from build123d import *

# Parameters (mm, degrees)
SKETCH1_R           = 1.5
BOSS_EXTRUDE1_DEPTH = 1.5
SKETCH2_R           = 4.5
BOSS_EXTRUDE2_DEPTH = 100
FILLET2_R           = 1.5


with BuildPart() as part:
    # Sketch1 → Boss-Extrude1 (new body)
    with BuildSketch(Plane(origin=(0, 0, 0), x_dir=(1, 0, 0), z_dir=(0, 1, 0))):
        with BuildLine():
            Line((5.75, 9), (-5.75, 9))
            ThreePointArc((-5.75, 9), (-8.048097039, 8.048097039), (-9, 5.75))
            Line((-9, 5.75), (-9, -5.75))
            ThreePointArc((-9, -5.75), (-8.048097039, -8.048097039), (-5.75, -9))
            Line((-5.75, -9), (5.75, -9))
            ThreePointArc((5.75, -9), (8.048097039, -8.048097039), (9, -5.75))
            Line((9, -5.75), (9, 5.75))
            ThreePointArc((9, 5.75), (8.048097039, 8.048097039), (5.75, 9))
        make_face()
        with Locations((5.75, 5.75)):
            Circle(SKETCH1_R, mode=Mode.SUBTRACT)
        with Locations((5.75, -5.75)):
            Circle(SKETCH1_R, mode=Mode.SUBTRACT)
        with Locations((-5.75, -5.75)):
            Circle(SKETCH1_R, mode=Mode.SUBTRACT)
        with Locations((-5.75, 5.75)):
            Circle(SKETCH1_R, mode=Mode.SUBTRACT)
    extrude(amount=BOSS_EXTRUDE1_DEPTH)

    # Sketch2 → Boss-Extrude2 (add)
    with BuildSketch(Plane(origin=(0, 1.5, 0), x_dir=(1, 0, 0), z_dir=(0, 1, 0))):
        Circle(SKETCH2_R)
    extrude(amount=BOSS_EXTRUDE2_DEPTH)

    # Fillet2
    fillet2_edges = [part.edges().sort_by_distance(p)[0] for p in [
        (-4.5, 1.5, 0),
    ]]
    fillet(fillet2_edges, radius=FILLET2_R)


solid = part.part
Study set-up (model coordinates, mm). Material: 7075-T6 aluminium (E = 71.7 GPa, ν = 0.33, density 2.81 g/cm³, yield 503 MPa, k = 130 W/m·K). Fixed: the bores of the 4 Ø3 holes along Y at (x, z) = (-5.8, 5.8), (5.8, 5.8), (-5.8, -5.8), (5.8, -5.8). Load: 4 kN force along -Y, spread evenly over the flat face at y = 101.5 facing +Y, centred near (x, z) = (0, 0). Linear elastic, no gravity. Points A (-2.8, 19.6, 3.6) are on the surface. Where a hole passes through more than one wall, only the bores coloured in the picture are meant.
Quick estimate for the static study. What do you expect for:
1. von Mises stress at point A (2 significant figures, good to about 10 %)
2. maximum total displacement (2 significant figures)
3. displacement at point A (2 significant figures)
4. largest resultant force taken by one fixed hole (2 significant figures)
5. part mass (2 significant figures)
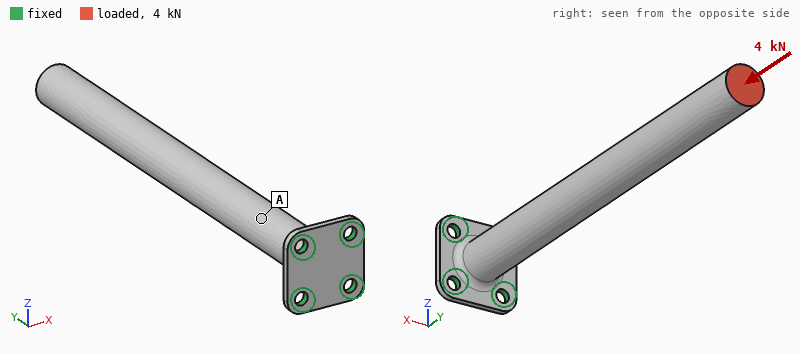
63 MPa
0.12 mm
0.043 mm
1.1 kN
19 g
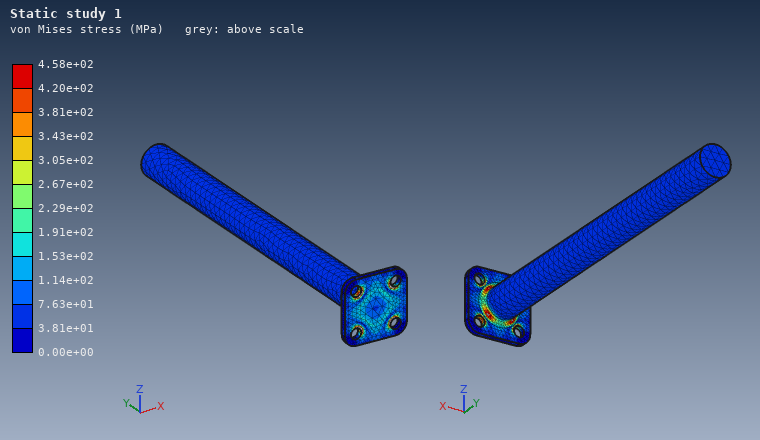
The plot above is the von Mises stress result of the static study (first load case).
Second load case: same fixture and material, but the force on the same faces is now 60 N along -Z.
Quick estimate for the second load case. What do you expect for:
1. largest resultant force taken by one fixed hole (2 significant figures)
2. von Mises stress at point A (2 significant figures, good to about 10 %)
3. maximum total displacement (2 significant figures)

320 N
54 MPa
1.1 mm
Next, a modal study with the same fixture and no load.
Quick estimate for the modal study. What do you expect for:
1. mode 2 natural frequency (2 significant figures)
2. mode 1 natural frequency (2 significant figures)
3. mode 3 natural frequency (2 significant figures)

550 Hz
550 Hz
3500 Hz
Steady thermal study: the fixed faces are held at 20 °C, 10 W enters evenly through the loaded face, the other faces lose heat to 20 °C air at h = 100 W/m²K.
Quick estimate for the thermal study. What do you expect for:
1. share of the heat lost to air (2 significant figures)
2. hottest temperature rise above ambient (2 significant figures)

72 %
63 K
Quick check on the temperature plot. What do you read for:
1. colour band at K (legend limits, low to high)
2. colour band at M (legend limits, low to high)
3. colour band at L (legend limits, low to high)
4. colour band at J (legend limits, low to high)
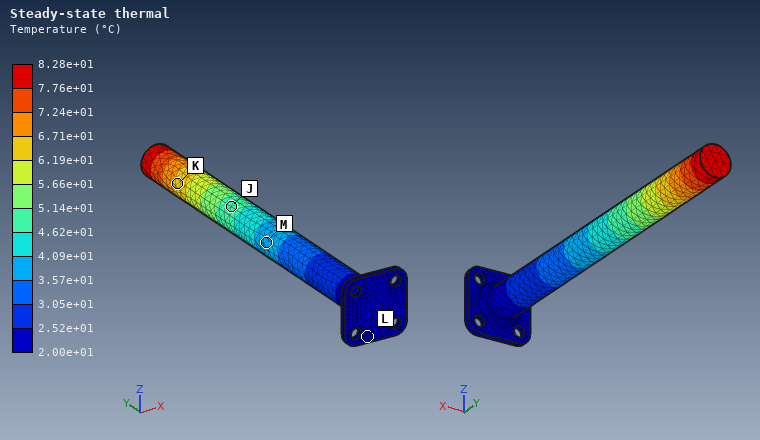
6.19e+01 to 6.71e+01 °C
3.57e+01 to 4.09e+01 °C
2.00e+01 to 2.52e+01 °C
4.62e+01 to 5.14e+01 °C
